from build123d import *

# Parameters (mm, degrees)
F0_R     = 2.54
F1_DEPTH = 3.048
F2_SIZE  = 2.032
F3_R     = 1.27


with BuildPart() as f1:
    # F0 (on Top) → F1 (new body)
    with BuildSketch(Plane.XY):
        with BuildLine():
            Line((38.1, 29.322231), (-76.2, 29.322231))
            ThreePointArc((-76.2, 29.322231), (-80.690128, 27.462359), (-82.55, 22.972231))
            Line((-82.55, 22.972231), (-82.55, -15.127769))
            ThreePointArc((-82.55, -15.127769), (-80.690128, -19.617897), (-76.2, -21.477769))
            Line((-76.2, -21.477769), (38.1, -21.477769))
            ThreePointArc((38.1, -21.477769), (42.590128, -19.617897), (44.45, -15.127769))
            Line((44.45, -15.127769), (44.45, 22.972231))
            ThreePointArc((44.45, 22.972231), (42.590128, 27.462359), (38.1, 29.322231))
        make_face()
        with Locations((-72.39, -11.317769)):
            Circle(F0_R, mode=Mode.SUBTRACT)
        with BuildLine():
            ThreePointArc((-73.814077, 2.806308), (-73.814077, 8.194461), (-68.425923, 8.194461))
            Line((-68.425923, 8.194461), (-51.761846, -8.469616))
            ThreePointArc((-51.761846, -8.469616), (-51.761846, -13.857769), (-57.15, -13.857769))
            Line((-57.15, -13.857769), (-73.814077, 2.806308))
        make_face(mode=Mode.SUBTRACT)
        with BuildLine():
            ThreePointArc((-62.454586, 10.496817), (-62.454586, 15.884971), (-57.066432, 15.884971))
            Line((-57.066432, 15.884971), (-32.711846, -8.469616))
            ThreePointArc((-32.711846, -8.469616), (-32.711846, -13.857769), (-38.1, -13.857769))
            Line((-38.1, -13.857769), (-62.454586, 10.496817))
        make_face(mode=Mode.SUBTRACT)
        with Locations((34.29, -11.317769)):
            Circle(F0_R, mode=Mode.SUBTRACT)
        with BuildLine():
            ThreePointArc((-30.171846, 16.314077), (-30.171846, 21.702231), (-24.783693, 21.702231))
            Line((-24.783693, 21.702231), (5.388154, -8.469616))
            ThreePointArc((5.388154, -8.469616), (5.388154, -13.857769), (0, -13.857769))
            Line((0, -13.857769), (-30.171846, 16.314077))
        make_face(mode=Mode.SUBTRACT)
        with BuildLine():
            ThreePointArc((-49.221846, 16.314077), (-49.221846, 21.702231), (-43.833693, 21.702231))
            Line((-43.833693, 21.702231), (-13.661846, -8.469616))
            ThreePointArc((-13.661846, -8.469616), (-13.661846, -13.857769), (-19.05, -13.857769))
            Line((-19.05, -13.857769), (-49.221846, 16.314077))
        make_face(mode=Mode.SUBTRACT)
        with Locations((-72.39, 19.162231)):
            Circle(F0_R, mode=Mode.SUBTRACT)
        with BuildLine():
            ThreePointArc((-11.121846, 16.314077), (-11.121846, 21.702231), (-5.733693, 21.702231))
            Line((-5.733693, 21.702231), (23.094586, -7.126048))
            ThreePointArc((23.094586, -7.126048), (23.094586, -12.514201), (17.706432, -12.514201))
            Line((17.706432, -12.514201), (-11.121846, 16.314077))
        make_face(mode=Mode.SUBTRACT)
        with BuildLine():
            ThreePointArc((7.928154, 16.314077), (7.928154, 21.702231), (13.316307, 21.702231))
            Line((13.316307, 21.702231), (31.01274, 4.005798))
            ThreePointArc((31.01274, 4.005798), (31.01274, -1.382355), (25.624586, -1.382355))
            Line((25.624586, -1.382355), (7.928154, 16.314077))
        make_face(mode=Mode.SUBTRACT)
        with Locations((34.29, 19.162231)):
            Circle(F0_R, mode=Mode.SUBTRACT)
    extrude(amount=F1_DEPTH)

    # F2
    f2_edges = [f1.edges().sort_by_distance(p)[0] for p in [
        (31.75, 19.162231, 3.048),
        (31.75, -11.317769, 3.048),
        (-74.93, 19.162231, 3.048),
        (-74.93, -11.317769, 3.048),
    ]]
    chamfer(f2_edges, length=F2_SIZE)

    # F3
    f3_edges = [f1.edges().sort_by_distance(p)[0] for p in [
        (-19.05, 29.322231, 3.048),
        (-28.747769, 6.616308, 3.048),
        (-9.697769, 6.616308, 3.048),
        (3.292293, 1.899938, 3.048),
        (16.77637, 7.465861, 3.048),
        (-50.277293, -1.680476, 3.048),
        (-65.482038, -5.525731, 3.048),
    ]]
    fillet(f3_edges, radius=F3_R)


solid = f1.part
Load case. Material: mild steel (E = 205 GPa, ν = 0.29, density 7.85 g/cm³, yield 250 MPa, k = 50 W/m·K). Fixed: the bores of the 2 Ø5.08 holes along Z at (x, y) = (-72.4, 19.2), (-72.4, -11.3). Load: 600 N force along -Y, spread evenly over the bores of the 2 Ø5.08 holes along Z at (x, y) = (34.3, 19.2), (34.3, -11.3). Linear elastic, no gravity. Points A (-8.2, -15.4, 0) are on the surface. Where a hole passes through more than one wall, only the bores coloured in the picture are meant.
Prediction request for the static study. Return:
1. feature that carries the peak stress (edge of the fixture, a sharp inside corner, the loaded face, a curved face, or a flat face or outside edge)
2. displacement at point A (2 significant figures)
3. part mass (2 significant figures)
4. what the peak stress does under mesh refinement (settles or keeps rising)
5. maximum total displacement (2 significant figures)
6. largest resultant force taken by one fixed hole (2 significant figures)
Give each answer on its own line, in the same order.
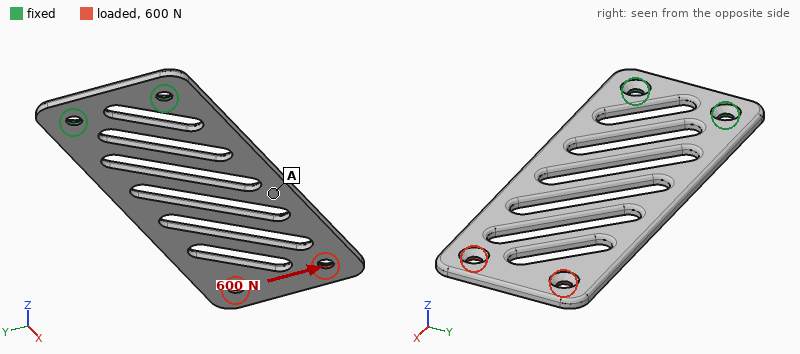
edge of the fixture
0.081 mm
100 g
keeps rising
0.26 mm
1.9 kN
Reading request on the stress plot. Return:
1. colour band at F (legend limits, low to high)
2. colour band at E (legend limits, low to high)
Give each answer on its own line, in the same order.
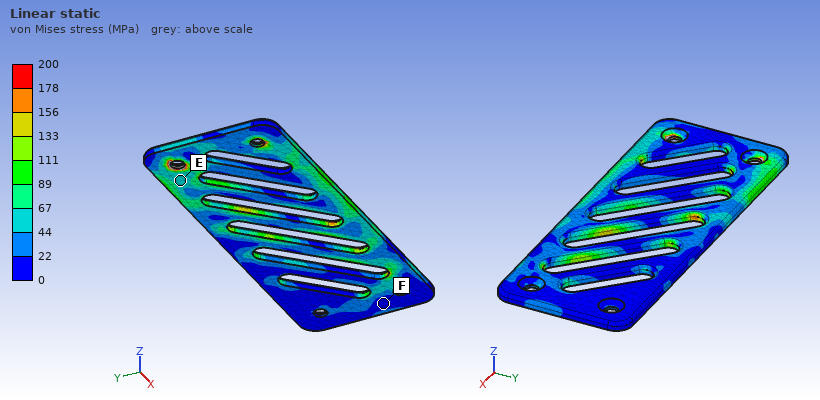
0 to 22 MPa
44 to 67 MPa
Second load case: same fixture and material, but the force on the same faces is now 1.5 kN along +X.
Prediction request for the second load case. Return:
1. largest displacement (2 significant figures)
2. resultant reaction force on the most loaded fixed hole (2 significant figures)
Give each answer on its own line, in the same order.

0.98 mm
780 N
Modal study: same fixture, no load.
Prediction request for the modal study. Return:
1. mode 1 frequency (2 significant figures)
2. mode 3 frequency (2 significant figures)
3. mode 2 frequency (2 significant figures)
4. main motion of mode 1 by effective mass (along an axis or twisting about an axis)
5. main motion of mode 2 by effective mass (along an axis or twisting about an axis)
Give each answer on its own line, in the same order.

140 Hz
910 Hz
620 Hz
along Z
twisting about X
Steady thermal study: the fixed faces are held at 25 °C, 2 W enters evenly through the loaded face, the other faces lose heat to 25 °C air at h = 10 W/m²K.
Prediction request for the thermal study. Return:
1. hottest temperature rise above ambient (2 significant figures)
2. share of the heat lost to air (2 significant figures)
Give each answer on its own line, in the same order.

32 K
72 %
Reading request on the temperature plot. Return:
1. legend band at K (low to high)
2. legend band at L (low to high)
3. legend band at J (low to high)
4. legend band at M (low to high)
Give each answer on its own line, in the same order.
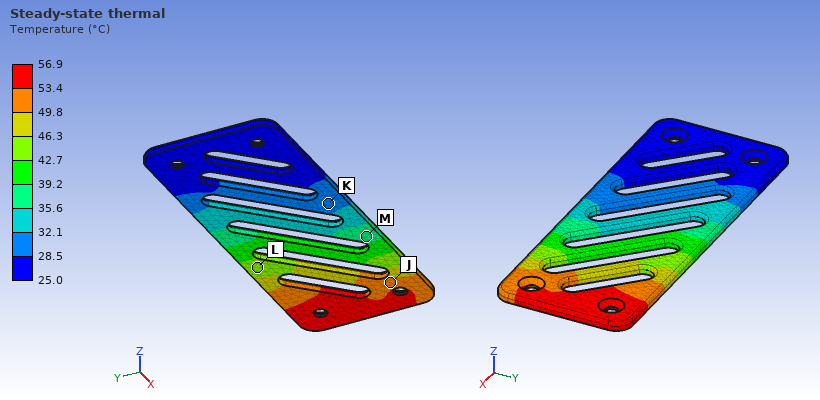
28.5 to 32.1 °C
42.7 to 46.3 °C
49.8 to 53.4 °C
35.6 to 39.2 °C
